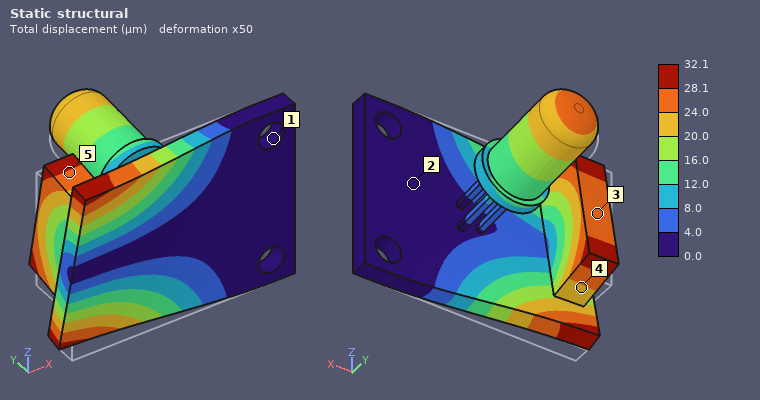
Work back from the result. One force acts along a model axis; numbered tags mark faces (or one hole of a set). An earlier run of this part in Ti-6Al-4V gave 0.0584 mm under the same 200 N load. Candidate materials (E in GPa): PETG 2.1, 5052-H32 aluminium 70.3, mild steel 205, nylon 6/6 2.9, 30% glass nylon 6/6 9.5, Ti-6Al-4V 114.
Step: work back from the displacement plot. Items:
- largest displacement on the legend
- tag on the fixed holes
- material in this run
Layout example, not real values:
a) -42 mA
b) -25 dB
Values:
a) 32.1 µm
b) 1
c) mild steel
